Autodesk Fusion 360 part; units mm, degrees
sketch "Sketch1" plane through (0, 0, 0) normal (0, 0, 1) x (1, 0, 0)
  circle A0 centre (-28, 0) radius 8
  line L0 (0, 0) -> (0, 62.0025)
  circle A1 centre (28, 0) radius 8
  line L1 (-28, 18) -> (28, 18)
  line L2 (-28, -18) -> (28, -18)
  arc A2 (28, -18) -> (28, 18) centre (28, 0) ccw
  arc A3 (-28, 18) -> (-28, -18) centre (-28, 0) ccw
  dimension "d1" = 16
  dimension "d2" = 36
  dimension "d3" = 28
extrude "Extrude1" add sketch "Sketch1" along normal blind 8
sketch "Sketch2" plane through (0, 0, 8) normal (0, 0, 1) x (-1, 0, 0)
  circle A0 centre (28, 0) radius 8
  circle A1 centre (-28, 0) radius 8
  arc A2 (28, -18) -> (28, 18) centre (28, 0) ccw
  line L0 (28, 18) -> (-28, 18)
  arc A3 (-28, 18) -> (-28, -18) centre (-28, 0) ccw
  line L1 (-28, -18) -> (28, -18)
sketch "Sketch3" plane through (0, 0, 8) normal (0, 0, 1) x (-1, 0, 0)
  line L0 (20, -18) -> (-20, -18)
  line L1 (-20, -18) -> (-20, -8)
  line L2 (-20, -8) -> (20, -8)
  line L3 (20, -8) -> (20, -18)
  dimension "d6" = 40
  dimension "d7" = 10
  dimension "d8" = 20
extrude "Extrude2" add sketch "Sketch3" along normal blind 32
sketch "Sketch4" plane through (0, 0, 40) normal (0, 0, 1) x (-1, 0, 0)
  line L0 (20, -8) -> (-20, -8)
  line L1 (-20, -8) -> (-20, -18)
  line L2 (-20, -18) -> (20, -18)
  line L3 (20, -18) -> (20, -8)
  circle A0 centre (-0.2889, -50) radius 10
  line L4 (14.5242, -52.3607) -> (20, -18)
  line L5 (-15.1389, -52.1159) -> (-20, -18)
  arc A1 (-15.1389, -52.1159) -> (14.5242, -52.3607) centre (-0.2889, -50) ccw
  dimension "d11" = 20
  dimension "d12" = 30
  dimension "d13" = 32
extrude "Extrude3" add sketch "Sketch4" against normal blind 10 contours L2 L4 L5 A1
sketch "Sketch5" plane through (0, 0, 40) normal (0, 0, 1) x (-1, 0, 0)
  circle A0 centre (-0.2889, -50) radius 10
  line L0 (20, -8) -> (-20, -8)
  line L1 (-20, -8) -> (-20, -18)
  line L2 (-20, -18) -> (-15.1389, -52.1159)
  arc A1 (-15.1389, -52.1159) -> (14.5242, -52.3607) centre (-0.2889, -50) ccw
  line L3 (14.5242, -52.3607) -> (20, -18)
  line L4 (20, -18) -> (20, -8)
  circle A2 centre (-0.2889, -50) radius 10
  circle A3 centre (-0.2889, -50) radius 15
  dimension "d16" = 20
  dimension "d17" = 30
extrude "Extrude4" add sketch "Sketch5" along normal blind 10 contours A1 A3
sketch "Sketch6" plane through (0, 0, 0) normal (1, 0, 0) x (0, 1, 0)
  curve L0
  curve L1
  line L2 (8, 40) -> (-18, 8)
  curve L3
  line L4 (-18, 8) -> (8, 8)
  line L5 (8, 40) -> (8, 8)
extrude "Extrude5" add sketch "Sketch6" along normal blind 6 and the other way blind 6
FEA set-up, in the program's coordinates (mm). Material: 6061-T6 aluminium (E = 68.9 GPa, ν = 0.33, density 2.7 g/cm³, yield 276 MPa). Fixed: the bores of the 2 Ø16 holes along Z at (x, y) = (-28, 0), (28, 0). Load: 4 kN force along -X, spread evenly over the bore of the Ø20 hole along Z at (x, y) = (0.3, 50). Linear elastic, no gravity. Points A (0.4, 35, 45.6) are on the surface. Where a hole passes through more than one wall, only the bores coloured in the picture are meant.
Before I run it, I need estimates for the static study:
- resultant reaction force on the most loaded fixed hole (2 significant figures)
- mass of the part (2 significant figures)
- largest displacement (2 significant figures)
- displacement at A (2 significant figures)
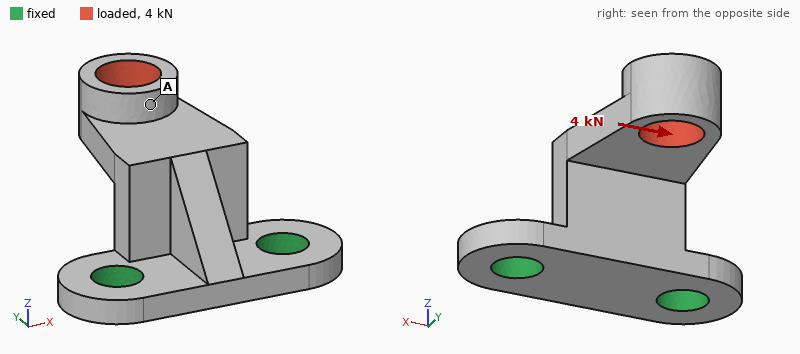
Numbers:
5.3 kN
150 g
0.42 mm
0.19 mm
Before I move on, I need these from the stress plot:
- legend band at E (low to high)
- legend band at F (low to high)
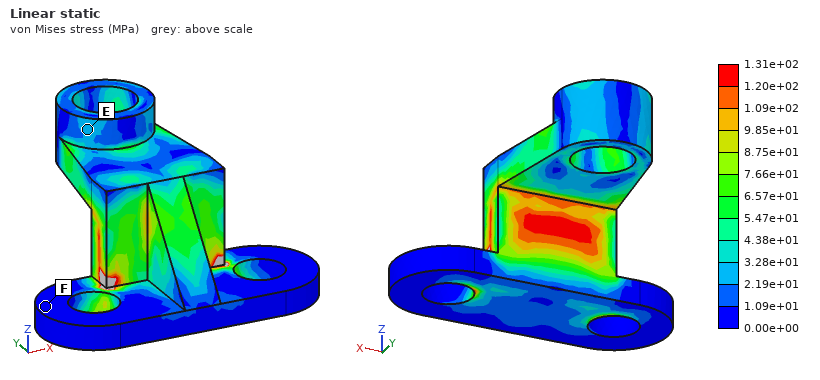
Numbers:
2.19e+01 to 3.28e+01 MPa
0.00e+00 to 1.09e+01 MPa
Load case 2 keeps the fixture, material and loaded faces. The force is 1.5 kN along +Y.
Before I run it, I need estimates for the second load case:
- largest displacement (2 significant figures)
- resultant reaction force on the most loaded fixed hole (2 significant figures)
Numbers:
0.20 mm
770 N
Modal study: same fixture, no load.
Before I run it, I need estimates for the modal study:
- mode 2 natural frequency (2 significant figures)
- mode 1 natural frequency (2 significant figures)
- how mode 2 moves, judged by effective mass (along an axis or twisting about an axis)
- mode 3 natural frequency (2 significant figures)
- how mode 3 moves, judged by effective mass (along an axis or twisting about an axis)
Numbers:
3300 Hz
2000 Hz
along X
5100 Hz
along Y
